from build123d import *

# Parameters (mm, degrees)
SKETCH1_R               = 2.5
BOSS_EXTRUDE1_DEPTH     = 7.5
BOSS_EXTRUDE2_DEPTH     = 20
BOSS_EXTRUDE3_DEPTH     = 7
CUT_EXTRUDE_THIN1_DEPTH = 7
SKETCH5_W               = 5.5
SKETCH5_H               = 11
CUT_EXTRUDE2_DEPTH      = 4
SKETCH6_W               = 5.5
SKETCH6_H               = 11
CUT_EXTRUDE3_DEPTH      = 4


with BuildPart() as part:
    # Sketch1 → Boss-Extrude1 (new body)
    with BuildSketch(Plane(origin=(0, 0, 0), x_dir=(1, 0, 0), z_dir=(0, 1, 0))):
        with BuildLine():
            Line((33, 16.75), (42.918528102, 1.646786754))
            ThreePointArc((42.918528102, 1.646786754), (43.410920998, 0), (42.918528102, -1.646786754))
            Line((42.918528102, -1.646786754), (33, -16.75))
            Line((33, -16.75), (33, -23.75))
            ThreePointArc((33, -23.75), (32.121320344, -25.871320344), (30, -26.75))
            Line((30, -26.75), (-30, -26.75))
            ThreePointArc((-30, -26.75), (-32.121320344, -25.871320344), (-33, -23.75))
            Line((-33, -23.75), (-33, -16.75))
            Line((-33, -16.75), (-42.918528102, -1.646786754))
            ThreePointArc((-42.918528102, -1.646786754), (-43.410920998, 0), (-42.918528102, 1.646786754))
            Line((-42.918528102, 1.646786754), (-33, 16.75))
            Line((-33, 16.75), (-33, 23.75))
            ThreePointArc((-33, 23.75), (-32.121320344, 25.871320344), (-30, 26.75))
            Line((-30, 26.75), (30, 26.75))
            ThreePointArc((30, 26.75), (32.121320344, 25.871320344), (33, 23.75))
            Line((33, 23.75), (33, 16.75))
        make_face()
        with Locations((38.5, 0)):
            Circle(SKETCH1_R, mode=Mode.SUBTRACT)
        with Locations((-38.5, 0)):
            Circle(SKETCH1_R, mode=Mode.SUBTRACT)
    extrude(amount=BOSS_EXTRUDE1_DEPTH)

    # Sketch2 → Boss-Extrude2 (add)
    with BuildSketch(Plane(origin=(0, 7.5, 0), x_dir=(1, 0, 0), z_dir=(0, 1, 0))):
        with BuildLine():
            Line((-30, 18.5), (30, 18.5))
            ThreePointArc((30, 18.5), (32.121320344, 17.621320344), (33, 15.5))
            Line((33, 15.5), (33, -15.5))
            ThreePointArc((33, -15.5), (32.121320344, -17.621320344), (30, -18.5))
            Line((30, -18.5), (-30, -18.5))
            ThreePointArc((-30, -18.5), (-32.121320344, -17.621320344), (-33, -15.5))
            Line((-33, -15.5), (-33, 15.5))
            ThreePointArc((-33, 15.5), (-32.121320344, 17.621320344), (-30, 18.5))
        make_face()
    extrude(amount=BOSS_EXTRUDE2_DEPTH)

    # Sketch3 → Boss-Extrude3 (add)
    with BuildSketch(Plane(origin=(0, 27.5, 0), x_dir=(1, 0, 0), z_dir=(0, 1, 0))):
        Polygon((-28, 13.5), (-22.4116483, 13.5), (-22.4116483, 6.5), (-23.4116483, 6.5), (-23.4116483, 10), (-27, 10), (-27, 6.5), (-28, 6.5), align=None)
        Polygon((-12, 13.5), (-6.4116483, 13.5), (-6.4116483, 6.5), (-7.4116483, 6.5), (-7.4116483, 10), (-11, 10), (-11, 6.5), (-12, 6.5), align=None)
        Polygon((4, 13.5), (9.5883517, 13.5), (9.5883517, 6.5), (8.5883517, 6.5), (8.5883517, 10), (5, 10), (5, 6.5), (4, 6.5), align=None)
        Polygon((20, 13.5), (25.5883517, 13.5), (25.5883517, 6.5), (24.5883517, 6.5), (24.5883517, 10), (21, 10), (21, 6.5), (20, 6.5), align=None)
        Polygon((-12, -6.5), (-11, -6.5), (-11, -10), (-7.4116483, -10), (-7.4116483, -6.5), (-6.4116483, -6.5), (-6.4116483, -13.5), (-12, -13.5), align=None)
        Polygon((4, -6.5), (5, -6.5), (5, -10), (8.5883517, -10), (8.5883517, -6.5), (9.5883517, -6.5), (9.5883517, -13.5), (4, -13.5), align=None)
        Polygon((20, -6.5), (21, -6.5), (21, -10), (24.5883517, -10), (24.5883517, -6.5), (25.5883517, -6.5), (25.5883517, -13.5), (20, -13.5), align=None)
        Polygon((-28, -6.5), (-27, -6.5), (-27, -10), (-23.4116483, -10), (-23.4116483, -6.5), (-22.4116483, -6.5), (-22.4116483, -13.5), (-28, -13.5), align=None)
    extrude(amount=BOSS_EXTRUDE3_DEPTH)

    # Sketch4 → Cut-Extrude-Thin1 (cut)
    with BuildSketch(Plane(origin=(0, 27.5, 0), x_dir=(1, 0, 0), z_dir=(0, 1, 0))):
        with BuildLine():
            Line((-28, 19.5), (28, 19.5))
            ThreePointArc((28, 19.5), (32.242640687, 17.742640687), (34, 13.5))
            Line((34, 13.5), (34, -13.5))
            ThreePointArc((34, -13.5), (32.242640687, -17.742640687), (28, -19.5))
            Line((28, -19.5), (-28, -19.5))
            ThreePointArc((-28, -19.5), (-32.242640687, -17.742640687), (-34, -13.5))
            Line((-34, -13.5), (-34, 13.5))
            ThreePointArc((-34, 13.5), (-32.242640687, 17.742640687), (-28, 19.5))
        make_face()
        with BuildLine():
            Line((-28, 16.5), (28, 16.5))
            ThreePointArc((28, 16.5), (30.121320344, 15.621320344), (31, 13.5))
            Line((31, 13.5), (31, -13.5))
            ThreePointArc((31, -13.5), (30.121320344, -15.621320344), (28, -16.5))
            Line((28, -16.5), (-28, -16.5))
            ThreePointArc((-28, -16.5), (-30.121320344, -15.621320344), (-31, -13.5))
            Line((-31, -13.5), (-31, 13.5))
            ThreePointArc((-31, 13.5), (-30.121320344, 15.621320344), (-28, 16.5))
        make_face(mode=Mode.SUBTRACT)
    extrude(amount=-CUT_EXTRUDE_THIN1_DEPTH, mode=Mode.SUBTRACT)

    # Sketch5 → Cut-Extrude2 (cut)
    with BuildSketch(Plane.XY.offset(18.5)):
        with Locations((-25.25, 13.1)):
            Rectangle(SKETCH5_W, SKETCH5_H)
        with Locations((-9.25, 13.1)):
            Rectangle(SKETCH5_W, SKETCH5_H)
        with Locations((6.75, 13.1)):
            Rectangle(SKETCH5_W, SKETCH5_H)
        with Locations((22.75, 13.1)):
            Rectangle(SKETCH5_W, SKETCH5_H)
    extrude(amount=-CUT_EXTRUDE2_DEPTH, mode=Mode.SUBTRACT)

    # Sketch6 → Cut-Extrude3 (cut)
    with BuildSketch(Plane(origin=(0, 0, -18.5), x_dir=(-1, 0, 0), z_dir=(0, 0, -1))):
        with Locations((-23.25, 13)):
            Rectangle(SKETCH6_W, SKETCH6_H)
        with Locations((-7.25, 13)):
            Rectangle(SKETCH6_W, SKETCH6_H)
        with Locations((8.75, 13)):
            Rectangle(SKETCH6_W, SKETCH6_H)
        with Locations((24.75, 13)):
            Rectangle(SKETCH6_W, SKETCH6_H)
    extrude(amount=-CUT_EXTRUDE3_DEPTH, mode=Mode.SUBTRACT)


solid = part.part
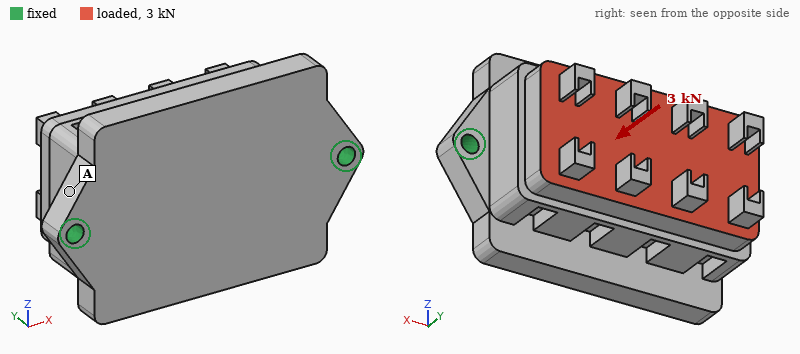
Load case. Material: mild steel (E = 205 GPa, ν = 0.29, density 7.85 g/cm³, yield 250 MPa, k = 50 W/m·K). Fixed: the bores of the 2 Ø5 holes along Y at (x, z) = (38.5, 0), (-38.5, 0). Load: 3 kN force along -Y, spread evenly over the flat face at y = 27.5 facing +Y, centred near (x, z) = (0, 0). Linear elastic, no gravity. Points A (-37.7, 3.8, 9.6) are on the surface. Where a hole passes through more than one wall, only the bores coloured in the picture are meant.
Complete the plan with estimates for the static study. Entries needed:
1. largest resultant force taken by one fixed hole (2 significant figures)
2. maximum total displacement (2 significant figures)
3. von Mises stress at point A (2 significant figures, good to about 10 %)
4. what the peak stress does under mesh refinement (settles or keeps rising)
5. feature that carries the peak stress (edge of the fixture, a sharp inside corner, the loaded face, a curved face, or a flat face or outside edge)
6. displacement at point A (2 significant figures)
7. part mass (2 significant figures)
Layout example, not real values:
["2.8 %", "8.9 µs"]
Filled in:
["1.7 kN", "3.2 µm", "11 MPa", "keeps rising", "edge of the fixture", "0.98 µm", "580 g"]
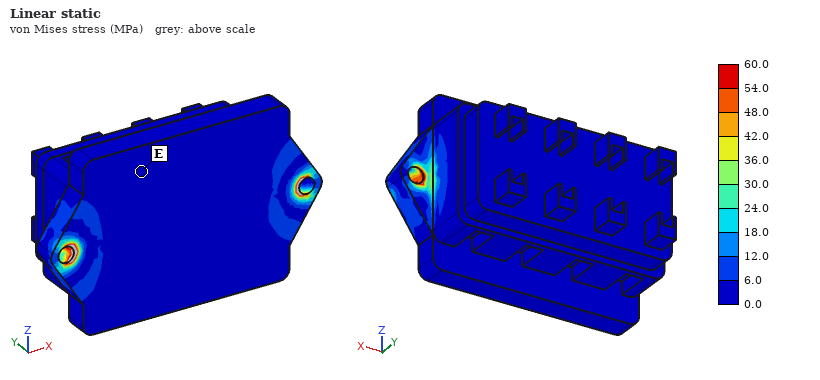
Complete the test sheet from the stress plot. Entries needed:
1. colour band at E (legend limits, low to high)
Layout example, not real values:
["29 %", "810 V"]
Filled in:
["0.0 to 6.0 MPa"]
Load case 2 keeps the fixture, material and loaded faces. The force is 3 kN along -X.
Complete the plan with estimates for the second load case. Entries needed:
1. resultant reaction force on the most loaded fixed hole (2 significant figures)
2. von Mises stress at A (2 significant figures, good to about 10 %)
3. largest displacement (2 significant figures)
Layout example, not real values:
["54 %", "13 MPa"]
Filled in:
["1.8 kN", "8.6 MPa", "2.4 µm"]
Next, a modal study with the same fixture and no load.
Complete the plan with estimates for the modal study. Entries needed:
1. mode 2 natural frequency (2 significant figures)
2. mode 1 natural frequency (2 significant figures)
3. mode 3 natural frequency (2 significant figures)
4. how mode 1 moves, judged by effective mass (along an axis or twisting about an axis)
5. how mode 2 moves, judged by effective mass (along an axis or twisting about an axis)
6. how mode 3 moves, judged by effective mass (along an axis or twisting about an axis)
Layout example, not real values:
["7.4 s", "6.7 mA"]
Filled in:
["7000 Hz", "2700 Hz", "10 kHz", "along Z", "along Y", "along Z"]
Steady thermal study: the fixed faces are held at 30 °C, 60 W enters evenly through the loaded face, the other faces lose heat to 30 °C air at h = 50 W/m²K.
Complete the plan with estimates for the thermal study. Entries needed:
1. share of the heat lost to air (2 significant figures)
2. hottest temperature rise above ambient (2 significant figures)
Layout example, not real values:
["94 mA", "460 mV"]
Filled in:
["35 %", "41 K"]
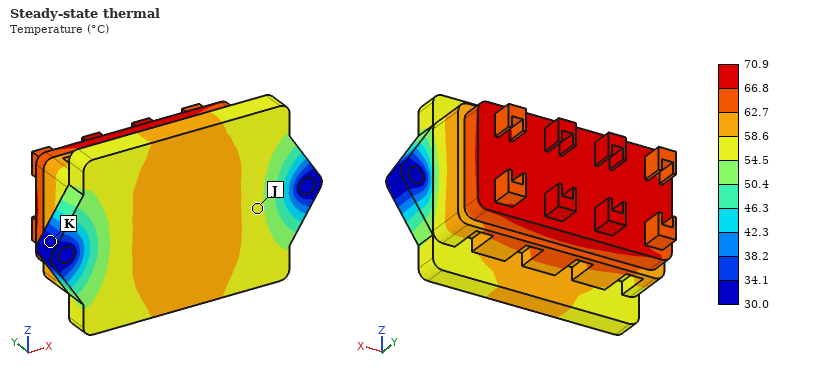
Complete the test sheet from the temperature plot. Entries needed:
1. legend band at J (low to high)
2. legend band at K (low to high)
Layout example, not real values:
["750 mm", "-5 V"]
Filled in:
["54.5 to 58.6 °C", "30.0 to 34.1 °C"]
